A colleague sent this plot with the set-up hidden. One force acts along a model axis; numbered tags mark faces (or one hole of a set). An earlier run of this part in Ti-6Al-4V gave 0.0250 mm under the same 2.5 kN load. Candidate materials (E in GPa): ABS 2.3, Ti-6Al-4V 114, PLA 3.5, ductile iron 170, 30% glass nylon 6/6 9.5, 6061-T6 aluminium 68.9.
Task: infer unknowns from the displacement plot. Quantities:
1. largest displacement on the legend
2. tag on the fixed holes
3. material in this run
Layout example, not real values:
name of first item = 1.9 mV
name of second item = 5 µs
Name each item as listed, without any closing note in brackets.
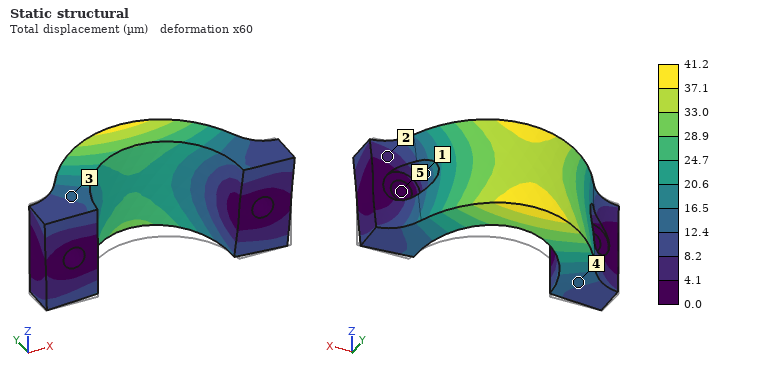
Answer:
largest displacement on the legend = 41.2 µm
tag on the fixed holes = 5
material in this run = 6061-T6 aluminium
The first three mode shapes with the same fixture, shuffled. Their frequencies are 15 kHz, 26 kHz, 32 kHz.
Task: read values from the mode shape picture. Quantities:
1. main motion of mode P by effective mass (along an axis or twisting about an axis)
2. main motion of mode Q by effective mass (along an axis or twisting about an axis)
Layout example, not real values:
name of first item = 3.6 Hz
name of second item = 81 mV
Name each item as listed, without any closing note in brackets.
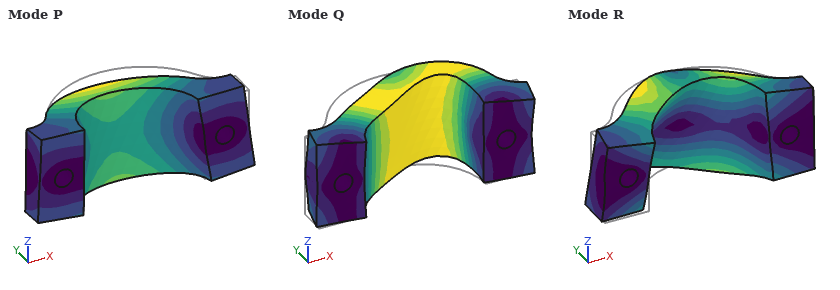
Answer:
main motion of mode P by effective mass = along Z
main motion of mode Q by effective mass = along X
